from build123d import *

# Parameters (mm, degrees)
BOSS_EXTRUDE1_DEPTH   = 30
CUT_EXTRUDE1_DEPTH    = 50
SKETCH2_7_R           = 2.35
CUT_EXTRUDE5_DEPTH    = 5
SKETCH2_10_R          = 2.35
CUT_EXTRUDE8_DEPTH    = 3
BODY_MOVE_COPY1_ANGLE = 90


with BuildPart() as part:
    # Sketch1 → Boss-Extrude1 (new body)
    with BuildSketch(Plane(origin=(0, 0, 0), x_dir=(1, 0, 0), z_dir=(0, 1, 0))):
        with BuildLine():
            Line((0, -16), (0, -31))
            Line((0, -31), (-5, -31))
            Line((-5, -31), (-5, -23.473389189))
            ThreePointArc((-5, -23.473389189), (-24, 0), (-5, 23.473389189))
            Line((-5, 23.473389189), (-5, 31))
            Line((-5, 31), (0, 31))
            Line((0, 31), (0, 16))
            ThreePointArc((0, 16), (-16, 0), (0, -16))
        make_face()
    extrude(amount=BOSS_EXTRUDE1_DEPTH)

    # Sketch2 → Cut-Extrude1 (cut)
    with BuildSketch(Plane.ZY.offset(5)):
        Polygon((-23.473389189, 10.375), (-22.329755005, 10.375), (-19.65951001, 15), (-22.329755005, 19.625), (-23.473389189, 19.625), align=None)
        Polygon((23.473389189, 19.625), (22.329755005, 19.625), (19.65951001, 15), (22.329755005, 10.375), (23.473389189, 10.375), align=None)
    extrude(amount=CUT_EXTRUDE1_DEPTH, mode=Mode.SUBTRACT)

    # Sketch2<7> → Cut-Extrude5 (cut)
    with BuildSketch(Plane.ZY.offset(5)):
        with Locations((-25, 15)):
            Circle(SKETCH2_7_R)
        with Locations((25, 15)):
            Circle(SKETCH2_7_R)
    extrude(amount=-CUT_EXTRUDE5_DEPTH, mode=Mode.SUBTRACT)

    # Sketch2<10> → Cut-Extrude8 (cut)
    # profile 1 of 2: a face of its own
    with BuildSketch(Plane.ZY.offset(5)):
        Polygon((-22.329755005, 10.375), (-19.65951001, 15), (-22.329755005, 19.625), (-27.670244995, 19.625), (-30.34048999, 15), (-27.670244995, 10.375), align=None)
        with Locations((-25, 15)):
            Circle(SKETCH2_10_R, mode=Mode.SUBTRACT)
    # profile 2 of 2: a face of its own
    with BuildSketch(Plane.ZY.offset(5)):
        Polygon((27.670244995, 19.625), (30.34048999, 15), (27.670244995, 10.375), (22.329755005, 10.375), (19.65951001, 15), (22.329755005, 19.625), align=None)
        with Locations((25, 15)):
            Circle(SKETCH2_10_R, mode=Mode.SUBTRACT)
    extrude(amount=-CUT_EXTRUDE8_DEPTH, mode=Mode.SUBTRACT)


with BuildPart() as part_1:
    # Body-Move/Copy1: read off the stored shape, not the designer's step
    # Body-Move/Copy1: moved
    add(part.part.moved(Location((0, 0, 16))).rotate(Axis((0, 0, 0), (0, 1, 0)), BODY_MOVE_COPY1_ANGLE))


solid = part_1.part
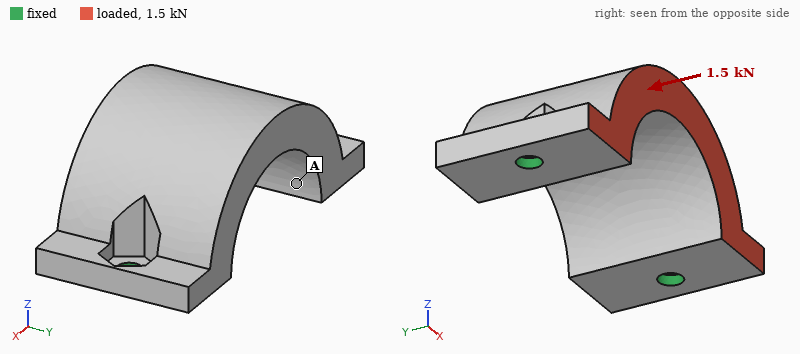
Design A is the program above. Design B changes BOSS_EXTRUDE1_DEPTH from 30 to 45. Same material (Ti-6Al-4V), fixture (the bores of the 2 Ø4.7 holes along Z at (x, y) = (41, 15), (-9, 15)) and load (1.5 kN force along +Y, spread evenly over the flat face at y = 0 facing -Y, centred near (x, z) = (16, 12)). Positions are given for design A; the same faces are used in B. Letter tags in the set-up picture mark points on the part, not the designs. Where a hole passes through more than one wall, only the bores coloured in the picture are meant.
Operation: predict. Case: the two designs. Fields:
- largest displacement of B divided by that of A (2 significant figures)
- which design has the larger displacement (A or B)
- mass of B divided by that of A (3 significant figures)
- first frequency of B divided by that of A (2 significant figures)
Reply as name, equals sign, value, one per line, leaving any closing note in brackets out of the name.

largest displacement of B divided by that of A = 1.3
which design has the larger displacement = B
mass of B divided by that of A = 1.52
first frequency of B divided by that of A = 0.65
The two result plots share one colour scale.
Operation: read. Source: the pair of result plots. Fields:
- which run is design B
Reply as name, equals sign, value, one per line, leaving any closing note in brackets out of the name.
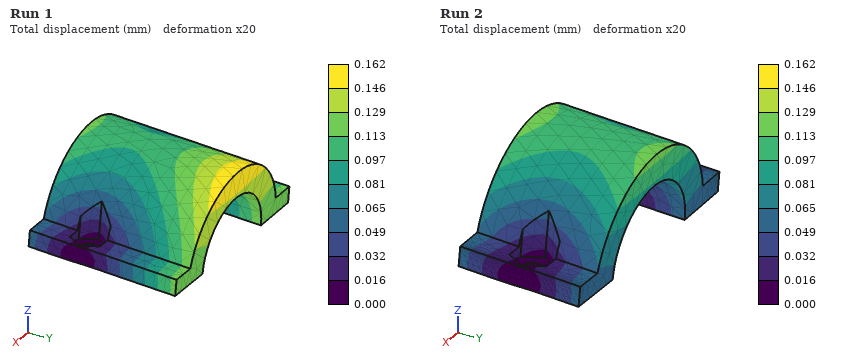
which run is design B = Run 1
